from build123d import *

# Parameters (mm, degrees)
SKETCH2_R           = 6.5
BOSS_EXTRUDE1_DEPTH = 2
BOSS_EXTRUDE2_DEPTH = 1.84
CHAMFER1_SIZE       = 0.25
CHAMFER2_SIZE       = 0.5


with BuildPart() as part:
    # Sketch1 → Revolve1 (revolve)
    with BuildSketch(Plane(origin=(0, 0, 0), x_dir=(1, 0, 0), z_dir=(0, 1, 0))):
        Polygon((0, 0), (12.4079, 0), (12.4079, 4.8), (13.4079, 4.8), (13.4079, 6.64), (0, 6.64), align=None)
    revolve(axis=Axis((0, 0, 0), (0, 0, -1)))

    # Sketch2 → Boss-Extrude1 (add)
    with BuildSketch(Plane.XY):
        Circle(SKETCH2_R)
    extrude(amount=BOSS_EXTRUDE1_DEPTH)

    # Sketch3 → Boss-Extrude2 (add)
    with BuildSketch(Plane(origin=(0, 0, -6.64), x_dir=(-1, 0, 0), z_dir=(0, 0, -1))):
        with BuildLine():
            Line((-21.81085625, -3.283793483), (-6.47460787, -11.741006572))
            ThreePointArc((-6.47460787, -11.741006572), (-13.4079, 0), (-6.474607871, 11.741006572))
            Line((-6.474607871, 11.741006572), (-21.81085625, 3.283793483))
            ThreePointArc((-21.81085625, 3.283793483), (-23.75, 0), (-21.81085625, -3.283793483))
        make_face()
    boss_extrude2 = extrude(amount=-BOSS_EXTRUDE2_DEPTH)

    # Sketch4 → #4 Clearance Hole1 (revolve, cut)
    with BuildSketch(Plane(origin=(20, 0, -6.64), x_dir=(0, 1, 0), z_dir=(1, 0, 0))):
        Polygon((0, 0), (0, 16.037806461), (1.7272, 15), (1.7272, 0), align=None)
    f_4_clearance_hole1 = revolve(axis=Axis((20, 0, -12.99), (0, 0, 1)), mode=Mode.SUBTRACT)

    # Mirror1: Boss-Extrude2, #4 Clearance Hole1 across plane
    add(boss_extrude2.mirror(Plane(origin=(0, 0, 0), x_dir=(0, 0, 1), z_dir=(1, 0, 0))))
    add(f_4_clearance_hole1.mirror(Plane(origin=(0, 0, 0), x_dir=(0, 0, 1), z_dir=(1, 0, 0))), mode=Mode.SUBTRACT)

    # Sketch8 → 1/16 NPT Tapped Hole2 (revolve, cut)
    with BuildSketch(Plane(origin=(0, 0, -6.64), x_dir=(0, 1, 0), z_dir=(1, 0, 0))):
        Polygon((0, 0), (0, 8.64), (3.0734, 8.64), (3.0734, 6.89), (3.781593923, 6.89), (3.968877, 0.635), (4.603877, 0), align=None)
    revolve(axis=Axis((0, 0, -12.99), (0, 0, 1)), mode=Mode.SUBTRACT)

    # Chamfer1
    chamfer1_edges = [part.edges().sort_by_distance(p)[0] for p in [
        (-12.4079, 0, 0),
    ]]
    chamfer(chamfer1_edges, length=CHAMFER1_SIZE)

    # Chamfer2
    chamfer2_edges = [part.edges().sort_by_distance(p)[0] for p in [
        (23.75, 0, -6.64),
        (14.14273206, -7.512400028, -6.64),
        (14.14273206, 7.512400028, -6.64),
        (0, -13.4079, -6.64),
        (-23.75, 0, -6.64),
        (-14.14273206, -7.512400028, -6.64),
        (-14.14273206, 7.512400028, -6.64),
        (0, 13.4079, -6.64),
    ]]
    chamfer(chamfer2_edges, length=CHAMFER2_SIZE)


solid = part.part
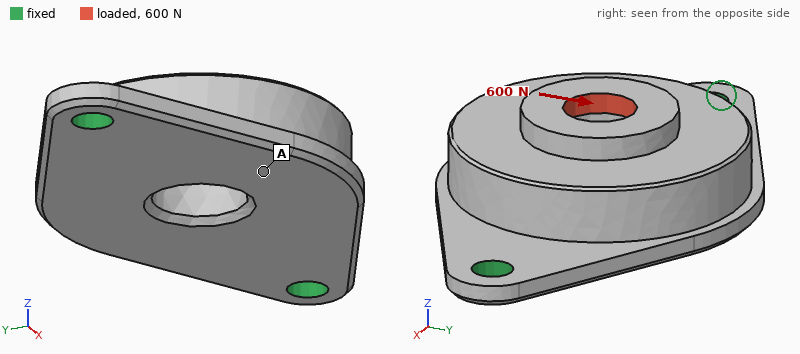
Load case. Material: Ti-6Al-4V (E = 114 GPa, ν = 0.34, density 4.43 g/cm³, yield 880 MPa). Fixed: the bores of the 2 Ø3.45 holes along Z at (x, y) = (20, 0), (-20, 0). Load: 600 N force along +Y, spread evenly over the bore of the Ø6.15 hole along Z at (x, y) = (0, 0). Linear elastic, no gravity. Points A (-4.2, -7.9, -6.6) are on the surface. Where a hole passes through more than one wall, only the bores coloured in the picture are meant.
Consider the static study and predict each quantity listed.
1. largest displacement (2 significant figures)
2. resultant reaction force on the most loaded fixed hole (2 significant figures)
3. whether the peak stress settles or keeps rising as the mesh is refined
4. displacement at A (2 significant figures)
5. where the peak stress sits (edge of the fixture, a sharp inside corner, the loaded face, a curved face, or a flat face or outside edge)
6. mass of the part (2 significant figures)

0.15 mm
300 N
keeps rising
0.086 mm
edge of the fixture
16 g
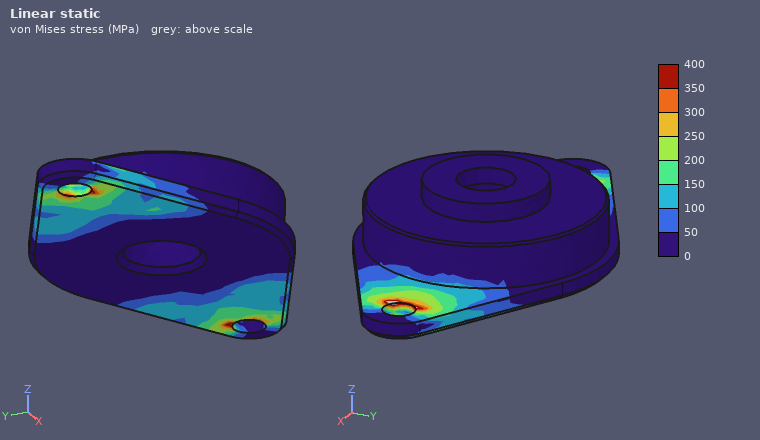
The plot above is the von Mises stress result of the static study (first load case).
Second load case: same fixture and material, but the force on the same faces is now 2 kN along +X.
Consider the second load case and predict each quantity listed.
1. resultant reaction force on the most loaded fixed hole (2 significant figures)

1.1 kN
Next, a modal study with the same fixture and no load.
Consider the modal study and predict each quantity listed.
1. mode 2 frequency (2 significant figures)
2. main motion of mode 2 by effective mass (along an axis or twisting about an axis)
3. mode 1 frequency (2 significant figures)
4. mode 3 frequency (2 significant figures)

6500 Hz
along Z
3500 Hz
14 kHz
